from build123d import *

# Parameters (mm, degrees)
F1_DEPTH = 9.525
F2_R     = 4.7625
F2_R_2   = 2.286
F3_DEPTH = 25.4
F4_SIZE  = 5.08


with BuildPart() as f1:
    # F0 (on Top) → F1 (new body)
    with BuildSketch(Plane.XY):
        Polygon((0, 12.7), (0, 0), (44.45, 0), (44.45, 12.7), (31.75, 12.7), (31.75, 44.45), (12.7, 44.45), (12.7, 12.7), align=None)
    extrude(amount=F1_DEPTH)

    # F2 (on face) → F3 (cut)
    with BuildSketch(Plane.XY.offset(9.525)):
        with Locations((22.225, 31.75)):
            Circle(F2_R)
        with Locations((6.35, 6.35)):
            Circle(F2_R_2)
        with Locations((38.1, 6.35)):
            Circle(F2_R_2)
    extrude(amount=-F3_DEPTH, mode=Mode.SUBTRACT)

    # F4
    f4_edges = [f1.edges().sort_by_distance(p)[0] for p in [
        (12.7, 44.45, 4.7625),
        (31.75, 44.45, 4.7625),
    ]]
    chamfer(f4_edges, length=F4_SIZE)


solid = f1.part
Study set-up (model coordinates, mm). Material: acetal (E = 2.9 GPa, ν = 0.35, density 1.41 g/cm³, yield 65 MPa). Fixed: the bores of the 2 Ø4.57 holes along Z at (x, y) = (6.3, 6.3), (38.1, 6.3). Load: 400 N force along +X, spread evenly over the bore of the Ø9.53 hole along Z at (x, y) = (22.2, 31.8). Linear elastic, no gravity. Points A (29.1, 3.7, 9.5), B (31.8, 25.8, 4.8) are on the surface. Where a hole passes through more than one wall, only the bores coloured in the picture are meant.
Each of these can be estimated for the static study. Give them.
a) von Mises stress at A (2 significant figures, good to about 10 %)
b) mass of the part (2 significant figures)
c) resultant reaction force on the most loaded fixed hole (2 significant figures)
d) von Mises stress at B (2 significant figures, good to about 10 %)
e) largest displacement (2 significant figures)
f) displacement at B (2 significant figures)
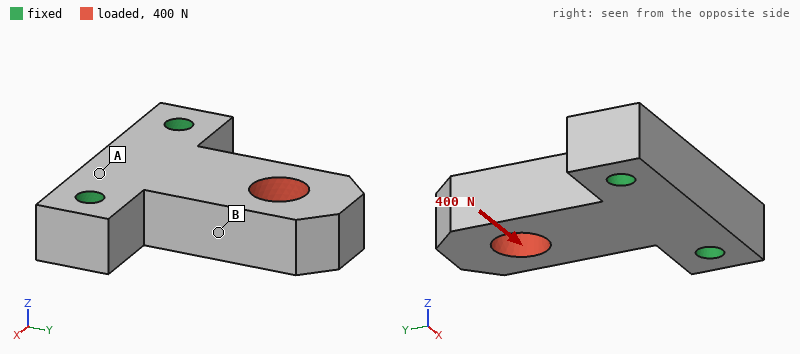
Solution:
2.0 MPa
14 g
410 N
7.8 MPa
0.32 mm
0.14 mm
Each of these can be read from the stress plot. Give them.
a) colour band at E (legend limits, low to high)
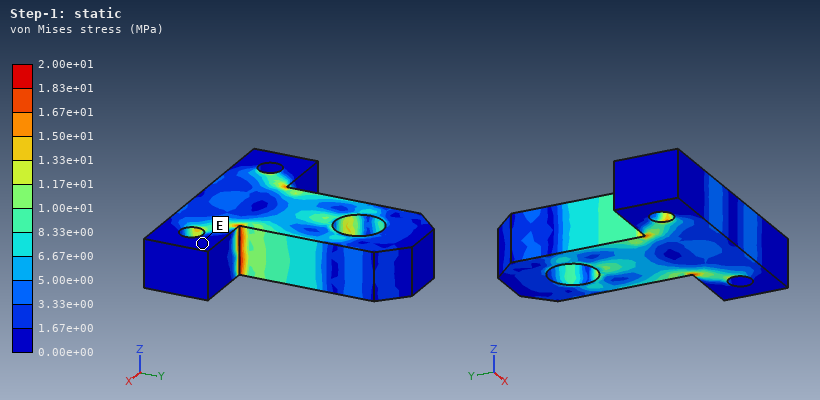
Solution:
0.00e+00 to 1.67e+00 MPa
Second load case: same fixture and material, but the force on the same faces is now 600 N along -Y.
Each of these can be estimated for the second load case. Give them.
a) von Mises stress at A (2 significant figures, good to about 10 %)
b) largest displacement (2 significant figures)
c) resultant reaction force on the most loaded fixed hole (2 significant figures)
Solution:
2.5 MPa
70 µm
320 N
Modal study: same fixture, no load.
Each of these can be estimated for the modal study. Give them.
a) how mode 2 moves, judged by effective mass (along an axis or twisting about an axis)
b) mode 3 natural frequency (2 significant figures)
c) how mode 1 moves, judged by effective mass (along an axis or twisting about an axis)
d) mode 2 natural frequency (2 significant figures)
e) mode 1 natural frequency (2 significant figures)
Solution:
along X
4700 Hz
along Z
2900 Hz
1300 Hz
